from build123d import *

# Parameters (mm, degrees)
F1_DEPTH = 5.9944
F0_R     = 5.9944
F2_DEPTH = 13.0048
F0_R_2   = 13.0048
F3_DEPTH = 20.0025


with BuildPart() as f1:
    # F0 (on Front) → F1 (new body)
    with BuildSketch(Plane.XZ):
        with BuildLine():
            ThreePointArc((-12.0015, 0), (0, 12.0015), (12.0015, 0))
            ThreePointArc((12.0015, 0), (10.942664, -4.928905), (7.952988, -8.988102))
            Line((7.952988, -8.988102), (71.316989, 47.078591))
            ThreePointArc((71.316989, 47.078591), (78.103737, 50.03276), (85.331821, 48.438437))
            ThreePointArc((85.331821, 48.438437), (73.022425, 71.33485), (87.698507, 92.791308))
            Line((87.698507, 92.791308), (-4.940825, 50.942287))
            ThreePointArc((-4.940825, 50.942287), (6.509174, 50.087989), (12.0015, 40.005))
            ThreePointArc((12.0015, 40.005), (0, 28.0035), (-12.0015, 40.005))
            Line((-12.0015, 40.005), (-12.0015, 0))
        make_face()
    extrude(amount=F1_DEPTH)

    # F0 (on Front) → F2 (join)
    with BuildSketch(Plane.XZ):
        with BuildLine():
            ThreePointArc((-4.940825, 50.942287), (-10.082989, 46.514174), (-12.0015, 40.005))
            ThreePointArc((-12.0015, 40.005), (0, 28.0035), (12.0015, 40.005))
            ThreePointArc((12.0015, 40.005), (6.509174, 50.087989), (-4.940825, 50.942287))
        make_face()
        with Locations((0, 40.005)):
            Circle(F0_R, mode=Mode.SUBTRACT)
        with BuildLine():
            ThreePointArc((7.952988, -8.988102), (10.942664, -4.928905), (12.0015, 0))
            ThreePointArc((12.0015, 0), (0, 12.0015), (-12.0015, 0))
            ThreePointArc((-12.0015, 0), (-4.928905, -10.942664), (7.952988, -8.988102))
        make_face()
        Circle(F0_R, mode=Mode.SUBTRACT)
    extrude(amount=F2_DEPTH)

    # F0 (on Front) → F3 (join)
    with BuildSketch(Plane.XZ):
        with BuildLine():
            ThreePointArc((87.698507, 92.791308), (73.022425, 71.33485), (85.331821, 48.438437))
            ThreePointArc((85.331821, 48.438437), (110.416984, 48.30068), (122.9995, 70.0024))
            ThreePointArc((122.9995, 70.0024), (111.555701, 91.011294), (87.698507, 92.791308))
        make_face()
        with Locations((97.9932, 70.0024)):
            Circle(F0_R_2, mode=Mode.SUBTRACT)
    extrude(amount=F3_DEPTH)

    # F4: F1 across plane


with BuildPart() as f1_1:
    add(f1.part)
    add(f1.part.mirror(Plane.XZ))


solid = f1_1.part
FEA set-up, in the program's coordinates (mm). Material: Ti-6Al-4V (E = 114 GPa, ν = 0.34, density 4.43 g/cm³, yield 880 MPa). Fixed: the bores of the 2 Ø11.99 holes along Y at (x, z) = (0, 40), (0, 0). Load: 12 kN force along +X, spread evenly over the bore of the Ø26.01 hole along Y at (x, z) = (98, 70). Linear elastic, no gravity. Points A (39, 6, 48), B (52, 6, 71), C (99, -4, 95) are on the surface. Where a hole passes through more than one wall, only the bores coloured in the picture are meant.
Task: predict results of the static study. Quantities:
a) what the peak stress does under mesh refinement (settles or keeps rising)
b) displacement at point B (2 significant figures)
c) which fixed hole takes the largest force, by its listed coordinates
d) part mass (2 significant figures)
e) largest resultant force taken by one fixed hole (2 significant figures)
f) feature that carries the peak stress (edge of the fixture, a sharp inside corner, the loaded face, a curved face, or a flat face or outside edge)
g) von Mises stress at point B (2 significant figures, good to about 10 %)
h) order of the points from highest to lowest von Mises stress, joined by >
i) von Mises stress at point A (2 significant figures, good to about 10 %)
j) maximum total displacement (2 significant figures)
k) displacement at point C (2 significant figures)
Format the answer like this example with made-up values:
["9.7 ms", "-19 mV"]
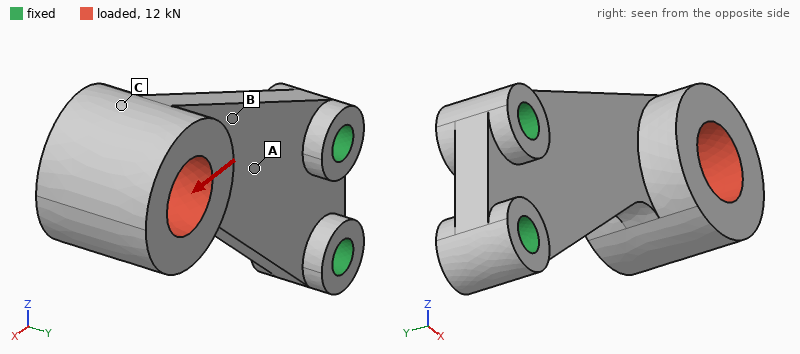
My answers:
["keeps rising", "0.077 mm", "(0, 40)", "530 g", "19 kN", "a sharp inside corner", "60 MPa", "B > A > C", "32 MPa", "0.21 mm", "0.19 mm"]
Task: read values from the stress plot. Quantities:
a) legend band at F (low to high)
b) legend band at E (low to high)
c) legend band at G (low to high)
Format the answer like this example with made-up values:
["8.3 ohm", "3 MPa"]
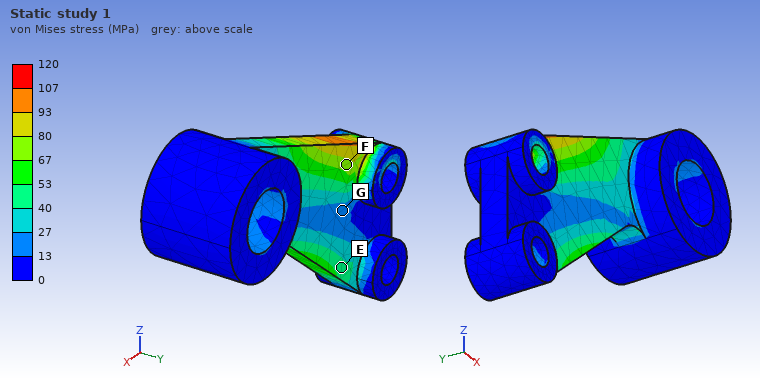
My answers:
["67 to 80 MPa", "40 to 53 MPa", "13 to 27 MPa"]
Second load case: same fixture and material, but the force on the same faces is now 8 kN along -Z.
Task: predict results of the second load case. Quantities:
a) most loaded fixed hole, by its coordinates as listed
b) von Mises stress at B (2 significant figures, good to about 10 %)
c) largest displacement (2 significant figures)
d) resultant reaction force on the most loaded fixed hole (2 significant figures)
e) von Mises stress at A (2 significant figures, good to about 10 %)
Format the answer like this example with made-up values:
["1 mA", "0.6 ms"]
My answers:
["(0, 0)", "78 MPa", "0.40 mm", "19 kN", "19 MPa"]
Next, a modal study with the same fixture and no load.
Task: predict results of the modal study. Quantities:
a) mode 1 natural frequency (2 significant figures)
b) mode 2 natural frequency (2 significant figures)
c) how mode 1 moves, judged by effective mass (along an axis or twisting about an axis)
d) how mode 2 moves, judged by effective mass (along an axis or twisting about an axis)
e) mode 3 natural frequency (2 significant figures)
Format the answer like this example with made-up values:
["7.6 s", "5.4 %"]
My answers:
["460 Hz", "1500 Hz", "along Y", "along Z", "1800 Hz"]
